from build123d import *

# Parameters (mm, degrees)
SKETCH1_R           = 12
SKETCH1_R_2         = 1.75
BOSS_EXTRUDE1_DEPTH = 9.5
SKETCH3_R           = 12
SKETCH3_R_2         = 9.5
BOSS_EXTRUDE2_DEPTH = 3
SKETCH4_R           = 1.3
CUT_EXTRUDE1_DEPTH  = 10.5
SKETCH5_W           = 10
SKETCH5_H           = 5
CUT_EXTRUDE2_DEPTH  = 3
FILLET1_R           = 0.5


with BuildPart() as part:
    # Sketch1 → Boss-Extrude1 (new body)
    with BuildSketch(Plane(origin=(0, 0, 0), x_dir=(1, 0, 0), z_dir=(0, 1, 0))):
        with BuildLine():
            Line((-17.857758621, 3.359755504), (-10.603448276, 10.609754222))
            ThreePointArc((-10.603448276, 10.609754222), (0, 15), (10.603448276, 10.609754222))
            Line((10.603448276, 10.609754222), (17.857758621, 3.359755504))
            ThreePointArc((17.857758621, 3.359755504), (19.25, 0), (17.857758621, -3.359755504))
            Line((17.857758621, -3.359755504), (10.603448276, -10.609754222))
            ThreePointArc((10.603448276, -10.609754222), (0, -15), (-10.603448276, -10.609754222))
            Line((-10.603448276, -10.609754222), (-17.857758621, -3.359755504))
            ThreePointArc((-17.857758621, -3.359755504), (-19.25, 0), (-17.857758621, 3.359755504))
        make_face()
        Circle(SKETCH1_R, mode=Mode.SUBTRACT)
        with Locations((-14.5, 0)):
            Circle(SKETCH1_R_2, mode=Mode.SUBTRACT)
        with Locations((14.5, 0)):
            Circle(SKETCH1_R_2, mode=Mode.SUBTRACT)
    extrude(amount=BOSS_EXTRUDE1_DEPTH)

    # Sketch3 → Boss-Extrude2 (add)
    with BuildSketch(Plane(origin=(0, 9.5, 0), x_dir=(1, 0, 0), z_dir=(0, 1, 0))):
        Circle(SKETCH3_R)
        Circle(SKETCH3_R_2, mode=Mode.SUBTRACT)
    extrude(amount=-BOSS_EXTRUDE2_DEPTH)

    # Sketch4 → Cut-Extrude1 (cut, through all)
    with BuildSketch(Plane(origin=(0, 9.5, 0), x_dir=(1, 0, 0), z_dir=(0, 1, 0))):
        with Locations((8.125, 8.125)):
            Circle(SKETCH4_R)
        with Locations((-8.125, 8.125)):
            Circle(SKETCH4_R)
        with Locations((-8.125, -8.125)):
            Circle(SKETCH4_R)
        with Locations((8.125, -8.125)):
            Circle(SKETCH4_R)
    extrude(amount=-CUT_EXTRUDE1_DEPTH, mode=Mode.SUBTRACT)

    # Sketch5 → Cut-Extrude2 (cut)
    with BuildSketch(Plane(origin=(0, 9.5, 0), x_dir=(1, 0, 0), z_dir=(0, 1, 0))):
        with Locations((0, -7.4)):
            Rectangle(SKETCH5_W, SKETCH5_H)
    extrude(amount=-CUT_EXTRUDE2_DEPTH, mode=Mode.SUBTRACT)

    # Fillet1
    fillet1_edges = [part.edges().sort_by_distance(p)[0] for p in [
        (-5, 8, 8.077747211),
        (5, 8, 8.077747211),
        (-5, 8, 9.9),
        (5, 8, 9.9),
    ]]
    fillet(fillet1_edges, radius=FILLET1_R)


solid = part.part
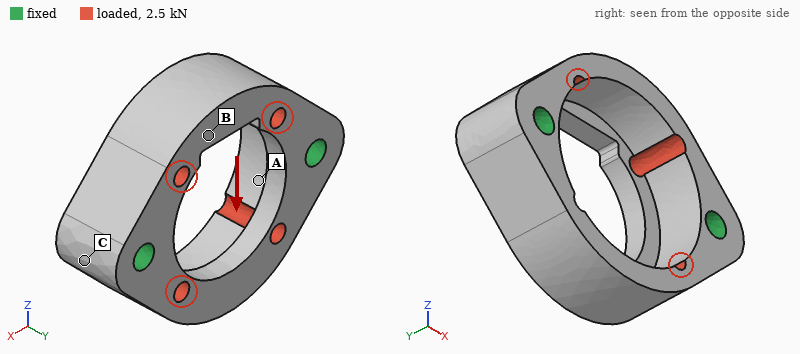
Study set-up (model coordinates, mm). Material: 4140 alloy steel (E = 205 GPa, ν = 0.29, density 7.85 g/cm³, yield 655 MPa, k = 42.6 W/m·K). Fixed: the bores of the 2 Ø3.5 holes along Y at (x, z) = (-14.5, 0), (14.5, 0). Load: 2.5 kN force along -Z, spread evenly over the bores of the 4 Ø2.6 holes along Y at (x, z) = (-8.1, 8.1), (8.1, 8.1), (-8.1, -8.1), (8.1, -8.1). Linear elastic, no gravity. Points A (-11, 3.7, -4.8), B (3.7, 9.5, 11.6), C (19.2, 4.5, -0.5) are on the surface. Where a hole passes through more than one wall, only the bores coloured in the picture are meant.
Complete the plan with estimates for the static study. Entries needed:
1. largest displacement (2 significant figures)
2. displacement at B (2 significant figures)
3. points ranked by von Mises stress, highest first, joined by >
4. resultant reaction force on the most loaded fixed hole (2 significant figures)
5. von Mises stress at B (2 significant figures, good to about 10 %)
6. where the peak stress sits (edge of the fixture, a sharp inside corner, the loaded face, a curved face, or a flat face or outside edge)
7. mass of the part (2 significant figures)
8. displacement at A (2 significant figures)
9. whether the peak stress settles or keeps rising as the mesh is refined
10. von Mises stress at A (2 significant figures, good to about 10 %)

2.3 µm
1.8 µm
A > B > C
1.3 kN
11 MPa
edge of the fixture
27 g
0.55 µm
keeps rising
27 MPa
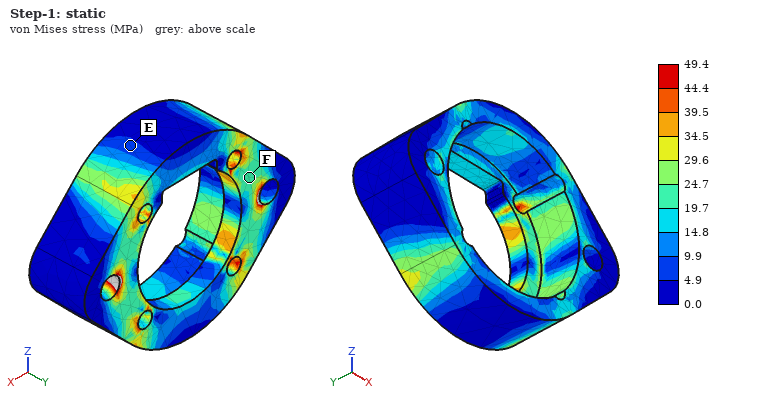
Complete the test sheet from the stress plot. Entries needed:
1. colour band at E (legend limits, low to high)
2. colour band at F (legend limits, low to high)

4.9 to 9.9 MPa
19.7 to 24.7 MPa
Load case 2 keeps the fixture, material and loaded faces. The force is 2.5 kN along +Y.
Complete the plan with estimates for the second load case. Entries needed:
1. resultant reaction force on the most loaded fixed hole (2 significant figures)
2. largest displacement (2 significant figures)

1.3 kN
7.2 µm
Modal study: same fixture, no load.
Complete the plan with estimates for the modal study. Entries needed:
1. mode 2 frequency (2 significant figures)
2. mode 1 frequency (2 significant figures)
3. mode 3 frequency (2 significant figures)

22 kHz
21 kHz
27 kHz
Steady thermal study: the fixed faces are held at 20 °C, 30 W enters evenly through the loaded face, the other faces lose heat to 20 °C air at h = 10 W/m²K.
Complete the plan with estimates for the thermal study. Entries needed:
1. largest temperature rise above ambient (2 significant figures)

46 K
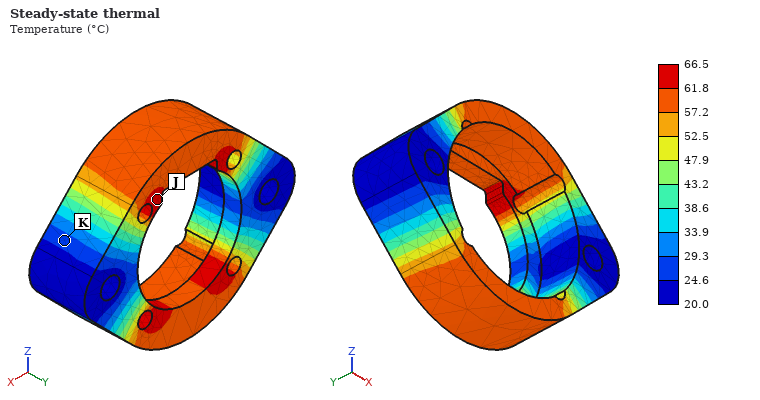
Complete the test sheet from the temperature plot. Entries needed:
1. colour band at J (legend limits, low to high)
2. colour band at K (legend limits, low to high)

61.8 to 66.5 °C
24.6 to 29.3 °C
